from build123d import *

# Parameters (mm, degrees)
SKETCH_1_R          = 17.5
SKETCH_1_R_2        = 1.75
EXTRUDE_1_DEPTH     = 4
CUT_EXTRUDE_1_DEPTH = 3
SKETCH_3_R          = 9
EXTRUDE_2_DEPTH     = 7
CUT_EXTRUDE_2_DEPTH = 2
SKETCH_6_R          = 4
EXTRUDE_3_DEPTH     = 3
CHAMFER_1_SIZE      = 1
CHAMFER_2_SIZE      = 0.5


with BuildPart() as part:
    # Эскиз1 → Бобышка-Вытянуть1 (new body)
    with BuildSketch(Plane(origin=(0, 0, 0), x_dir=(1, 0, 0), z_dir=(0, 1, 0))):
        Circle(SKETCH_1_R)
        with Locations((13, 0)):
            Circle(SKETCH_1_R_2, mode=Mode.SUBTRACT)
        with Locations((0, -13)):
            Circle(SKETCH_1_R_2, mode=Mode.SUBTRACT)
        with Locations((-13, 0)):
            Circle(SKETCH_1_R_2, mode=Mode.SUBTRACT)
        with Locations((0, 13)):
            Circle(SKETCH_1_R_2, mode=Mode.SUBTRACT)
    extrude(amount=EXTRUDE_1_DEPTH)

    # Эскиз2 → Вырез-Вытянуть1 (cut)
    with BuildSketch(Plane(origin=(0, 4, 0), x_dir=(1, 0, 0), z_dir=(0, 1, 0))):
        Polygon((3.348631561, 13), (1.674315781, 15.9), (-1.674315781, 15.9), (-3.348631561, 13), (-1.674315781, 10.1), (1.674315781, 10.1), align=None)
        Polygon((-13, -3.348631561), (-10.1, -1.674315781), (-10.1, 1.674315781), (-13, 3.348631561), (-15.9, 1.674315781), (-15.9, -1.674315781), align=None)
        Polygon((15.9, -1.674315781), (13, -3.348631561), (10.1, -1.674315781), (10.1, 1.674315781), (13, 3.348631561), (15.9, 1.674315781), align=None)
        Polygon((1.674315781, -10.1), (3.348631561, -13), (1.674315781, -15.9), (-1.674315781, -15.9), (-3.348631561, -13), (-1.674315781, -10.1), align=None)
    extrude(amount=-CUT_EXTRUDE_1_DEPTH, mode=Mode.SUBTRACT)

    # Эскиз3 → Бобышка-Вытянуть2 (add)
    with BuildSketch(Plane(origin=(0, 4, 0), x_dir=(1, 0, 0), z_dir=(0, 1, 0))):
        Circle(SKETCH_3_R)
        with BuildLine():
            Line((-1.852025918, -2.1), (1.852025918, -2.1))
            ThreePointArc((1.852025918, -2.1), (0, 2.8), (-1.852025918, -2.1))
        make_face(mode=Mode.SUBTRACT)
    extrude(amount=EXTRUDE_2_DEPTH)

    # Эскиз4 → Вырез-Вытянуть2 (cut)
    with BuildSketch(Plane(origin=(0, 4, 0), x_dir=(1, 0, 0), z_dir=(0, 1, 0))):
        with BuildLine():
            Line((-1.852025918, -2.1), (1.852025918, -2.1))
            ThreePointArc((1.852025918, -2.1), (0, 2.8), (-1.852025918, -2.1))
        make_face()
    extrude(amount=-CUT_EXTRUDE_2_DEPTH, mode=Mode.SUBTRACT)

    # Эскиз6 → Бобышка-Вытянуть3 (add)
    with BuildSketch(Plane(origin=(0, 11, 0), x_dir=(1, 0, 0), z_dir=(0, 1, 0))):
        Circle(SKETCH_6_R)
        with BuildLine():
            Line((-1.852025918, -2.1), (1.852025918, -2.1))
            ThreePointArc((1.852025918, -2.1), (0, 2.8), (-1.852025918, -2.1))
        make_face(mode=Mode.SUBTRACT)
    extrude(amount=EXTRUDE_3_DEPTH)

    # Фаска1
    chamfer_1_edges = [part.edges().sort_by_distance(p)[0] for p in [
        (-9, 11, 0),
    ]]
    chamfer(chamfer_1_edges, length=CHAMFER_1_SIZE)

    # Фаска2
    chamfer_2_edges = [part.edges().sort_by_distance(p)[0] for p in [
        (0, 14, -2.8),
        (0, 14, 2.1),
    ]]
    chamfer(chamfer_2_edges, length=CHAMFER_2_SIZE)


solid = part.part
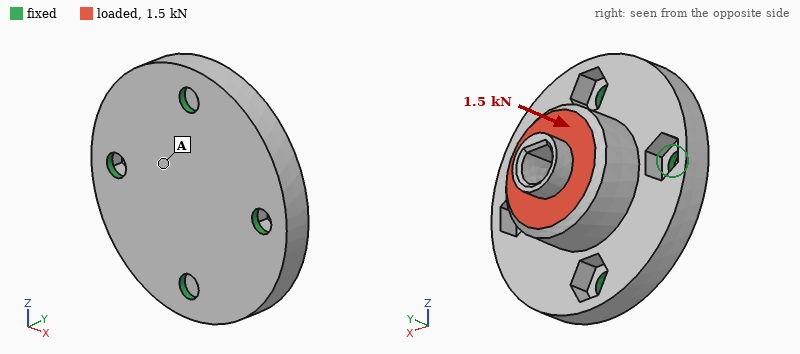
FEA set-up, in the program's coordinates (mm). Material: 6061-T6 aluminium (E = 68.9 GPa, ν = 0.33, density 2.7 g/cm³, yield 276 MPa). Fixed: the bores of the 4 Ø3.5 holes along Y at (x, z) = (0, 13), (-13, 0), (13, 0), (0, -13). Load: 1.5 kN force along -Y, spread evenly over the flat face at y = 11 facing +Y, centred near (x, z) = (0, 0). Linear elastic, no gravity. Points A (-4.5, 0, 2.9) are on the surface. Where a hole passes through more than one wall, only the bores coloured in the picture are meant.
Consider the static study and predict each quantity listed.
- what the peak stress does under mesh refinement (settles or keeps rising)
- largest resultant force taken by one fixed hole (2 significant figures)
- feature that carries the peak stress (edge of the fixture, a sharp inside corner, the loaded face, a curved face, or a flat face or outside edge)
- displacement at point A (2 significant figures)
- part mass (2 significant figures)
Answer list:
keeps rising
440 N
edge of the fixture
7.4 µm
14 g
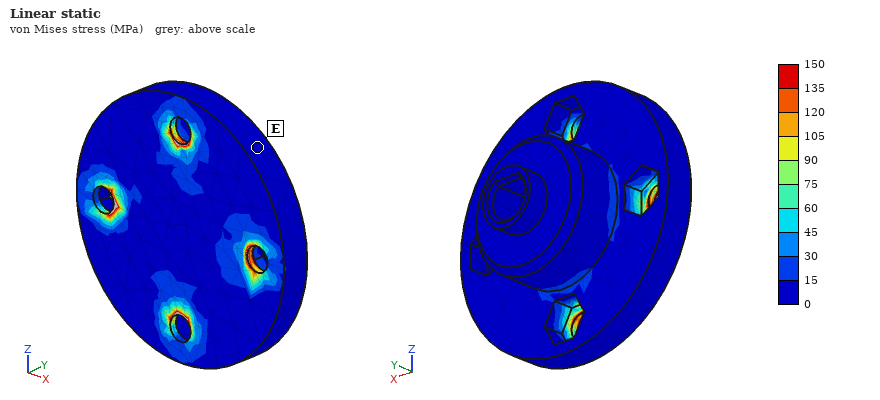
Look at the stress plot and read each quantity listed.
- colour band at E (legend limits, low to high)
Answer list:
0 to 15 MPa
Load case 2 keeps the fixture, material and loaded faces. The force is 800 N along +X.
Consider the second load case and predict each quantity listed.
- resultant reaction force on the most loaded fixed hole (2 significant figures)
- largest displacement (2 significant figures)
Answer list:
450 N
8.7 µm
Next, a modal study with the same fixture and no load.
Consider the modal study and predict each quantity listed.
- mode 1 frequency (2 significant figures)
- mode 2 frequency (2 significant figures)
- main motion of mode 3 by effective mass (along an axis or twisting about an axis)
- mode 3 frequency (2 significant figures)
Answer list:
22 kHz
22 kHz
along Y
23 kHz
